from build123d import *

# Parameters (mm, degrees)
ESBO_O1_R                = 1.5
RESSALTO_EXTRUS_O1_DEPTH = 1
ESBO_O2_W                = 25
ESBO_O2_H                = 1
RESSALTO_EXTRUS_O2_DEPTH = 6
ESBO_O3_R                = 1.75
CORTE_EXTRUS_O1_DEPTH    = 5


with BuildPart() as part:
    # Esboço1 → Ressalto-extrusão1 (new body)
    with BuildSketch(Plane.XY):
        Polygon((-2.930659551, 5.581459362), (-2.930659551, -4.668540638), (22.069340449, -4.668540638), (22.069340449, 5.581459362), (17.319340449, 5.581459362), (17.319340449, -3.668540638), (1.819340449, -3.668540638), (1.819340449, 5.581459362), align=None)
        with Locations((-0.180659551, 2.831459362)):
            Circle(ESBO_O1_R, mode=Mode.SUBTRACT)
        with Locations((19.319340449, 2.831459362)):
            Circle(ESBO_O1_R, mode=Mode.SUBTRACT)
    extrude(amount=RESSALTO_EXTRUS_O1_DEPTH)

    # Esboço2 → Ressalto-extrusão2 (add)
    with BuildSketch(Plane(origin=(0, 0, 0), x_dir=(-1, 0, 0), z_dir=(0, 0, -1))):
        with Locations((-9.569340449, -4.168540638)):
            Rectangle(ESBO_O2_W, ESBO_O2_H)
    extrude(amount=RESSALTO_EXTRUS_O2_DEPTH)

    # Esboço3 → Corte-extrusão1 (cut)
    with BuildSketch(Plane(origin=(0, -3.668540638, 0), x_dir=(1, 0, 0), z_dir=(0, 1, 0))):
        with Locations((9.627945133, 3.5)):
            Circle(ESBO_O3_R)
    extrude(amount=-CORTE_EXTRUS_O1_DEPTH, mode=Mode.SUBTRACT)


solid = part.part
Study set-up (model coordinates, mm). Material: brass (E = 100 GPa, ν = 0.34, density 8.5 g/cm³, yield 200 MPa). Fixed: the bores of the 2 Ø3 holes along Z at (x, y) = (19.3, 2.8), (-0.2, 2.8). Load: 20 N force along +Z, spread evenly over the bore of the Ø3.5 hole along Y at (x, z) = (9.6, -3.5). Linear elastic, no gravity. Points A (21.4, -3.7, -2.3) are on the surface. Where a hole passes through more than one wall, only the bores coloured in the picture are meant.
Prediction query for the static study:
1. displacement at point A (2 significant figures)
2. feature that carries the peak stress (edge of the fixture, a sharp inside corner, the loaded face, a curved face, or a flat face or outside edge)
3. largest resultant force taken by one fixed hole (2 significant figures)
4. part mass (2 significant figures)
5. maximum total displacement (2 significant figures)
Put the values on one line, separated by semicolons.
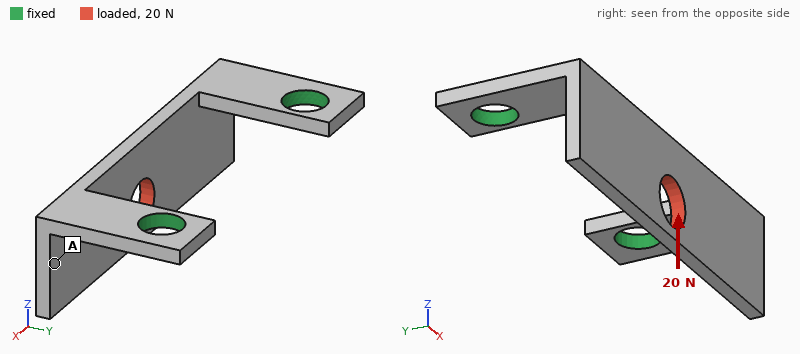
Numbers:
18 µm; a flat face or outside edge; 10 N; 2.0 g; 33 µm
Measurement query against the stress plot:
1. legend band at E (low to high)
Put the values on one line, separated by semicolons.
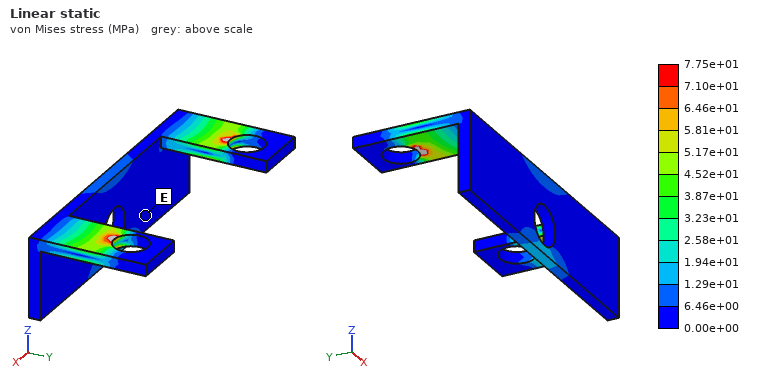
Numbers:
0.00e+00 to 6.46e+00 MPa
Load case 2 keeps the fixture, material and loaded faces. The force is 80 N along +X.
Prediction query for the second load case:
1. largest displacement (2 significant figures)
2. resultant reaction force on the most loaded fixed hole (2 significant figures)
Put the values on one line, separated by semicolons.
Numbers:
30 µm; 43 N
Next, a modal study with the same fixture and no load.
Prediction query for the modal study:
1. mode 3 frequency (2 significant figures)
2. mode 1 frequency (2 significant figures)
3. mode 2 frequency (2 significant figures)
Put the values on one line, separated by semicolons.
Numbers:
8100 Hz; 3200 Hz; 6000 Hz
